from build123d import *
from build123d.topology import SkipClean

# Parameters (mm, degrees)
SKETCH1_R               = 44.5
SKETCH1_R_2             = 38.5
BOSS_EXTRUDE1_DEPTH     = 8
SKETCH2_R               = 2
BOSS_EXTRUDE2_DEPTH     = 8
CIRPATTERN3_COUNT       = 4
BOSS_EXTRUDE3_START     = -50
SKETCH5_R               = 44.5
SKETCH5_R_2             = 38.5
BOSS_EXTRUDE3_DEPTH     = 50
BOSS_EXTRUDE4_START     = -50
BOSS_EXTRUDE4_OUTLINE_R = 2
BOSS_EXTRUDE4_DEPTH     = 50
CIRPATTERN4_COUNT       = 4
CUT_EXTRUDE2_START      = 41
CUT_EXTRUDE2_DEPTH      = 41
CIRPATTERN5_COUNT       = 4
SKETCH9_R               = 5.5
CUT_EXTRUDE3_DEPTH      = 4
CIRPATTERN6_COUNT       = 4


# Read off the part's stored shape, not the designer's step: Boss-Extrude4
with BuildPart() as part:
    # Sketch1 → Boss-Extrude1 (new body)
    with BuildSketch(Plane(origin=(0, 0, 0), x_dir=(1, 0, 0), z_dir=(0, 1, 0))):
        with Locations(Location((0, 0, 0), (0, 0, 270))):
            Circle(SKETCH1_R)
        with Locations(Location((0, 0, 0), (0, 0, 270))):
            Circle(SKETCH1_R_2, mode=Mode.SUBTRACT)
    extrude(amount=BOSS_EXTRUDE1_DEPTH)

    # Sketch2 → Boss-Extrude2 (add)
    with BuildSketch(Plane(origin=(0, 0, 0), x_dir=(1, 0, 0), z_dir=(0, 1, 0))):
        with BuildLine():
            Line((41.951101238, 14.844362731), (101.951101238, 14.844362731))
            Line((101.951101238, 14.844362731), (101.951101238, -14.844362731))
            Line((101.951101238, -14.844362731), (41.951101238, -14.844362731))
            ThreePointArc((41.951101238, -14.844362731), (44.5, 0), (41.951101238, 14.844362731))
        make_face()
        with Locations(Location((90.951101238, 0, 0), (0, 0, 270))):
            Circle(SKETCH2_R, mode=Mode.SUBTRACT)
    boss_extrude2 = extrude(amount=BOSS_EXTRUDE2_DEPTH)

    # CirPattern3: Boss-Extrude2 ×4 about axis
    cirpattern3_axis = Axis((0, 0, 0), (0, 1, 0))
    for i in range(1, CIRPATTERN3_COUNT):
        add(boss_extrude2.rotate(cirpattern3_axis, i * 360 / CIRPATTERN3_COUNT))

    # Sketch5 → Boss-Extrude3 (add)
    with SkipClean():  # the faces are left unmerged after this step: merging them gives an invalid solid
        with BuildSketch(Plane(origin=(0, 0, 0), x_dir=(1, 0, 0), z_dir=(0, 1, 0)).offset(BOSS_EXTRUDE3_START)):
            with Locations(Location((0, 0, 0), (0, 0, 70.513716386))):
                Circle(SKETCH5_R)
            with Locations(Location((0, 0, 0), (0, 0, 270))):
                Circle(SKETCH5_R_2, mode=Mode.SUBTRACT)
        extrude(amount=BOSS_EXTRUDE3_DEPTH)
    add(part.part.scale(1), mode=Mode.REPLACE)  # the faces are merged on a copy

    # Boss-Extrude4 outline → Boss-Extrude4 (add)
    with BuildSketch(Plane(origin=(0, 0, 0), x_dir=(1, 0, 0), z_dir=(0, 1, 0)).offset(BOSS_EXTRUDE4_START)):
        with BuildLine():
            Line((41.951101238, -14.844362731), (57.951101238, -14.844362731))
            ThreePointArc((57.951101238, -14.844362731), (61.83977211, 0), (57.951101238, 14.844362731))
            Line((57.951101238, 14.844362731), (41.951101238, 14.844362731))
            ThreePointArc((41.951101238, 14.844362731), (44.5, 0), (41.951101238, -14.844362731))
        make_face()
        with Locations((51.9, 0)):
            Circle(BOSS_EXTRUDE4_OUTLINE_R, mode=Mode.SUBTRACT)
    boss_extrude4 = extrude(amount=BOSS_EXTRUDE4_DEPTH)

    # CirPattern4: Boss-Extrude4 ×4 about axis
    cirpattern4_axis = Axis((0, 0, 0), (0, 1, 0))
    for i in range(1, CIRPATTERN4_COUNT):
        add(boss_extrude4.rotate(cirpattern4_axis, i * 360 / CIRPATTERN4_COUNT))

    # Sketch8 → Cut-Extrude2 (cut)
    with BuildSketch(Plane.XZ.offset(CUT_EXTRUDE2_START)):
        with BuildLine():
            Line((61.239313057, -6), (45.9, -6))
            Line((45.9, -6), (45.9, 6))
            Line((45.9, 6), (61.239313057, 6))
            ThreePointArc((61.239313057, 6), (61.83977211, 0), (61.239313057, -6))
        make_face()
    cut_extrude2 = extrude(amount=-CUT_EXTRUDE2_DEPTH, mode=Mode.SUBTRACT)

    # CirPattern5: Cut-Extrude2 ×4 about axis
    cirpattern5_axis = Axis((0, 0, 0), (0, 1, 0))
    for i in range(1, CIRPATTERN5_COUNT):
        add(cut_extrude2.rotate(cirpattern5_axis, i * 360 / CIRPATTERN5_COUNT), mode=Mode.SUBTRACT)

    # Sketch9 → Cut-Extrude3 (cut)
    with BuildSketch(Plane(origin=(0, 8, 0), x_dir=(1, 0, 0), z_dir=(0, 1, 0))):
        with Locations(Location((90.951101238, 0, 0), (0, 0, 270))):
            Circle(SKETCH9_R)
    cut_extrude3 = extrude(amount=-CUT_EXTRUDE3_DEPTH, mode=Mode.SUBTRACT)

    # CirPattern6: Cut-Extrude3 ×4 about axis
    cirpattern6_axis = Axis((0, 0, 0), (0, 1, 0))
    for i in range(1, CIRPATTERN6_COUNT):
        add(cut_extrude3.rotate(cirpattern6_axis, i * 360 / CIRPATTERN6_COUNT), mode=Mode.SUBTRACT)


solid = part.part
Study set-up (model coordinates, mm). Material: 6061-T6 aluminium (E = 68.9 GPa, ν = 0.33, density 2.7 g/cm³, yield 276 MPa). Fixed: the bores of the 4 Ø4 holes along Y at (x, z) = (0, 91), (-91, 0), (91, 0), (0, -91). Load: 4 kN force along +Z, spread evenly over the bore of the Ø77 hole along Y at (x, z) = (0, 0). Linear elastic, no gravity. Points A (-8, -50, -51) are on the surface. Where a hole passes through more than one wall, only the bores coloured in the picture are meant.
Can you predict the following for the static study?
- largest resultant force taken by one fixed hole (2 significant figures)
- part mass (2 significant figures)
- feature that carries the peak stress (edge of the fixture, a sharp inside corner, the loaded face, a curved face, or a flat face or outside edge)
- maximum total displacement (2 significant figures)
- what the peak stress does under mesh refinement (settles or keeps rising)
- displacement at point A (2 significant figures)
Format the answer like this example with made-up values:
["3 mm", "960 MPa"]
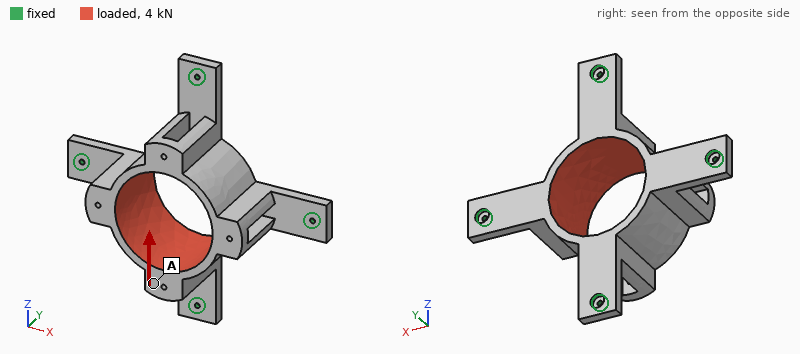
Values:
["2.0 kN", "580 g", "edge of the fixture", "79 µm", "keeps rising", "74 µm"]
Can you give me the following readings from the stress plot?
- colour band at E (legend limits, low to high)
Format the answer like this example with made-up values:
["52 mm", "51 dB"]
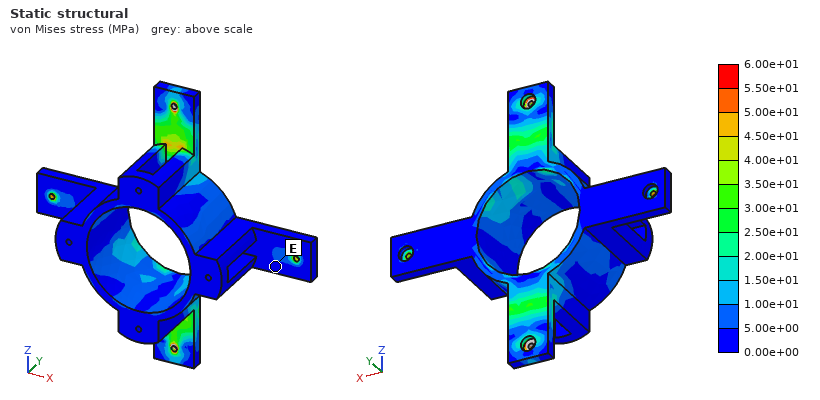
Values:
["0.00e+00 to 5.00e+00 MPa"]
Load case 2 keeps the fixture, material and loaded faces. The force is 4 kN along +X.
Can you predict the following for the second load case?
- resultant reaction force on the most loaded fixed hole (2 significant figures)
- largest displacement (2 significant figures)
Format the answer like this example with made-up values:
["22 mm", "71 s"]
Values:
["2.0 kN", "79 µm"]
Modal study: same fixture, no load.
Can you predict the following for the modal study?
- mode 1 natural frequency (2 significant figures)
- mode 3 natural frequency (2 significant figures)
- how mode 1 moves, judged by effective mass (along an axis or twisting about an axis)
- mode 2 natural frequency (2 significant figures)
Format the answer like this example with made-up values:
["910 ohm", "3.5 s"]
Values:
["1300 Hz", "1700 Hz", "along Y", "1700 Hz"]
